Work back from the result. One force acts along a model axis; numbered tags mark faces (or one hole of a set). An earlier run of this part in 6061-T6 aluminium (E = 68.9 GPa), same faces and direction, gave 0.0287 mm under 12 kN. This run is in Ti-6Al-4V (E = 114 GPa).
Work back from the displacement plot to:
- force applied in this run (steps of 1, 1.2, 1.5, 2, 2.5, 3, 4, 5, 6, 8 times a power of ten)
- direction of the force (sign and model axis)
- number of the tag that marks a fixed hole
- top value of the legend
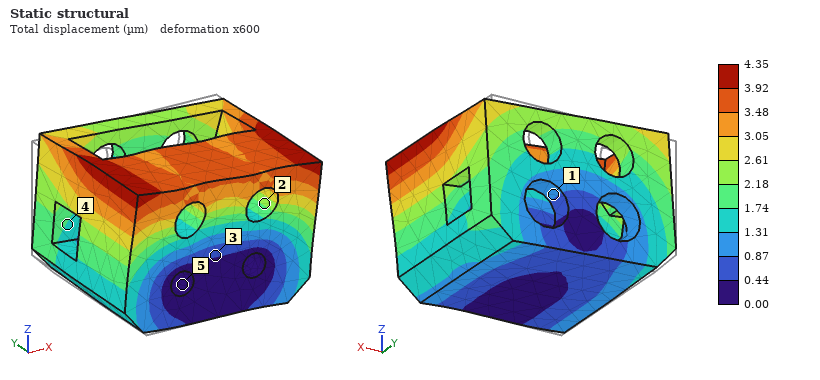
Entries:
3 kN
+X
5
4.35 µm
